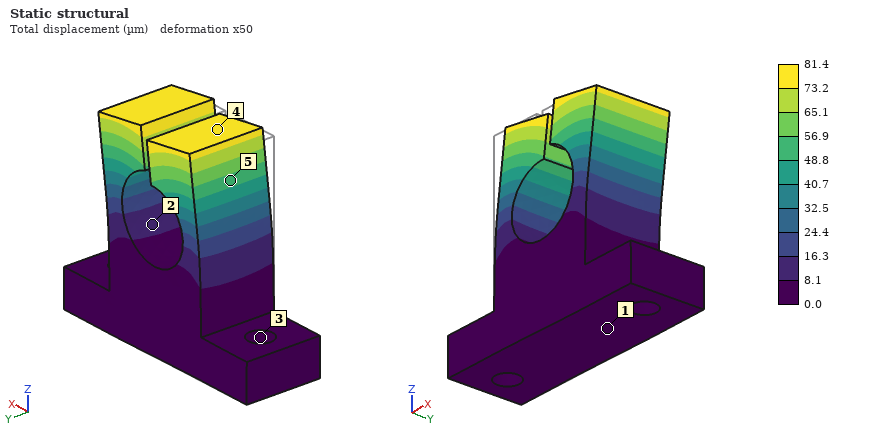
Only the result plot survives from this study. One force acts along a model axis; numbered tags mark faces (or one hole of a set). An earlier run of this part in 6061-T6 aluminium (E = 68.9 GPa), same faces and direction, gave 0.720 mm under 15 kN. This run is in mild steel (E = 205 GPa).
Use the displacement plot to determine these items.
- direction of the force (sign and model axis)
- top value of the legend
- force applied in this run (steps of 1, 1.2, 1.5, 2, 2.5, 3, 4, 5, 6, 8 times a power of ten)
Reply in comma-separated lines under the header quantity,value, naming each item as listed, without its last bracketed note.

quantity,value
direction of the force,+X
top value of the legend,81.4 µm
force applied in this run,5 kN
